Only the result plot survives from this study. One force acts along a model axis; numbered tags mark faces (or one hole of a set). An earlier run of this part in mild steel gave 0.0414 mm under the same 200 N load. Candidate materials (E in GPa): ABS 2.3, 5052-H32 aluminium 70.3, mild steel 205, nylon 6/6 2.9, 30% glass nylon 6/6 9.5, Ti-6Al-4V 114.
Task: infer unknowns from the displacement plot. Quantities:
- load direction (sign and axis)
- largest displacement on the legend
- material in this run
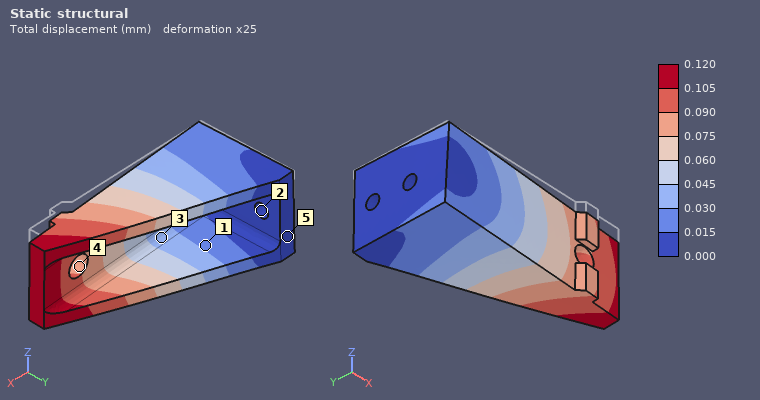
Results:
-Z
0.120 mm
5052-H32 aluminium
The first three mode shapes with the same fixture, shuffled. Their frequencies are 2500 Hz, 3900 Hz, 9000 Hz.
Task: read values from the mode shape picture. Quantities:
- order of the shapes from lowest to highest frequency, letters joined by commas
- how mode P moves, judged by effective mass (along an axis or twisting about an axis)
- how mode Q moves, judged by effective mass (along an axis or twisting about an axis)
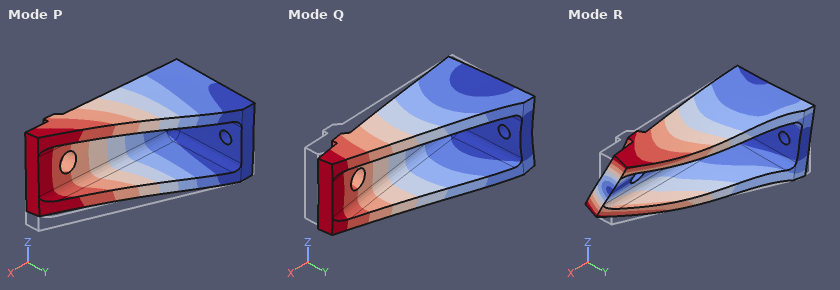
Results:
P, Q, R
along Z
along Y
